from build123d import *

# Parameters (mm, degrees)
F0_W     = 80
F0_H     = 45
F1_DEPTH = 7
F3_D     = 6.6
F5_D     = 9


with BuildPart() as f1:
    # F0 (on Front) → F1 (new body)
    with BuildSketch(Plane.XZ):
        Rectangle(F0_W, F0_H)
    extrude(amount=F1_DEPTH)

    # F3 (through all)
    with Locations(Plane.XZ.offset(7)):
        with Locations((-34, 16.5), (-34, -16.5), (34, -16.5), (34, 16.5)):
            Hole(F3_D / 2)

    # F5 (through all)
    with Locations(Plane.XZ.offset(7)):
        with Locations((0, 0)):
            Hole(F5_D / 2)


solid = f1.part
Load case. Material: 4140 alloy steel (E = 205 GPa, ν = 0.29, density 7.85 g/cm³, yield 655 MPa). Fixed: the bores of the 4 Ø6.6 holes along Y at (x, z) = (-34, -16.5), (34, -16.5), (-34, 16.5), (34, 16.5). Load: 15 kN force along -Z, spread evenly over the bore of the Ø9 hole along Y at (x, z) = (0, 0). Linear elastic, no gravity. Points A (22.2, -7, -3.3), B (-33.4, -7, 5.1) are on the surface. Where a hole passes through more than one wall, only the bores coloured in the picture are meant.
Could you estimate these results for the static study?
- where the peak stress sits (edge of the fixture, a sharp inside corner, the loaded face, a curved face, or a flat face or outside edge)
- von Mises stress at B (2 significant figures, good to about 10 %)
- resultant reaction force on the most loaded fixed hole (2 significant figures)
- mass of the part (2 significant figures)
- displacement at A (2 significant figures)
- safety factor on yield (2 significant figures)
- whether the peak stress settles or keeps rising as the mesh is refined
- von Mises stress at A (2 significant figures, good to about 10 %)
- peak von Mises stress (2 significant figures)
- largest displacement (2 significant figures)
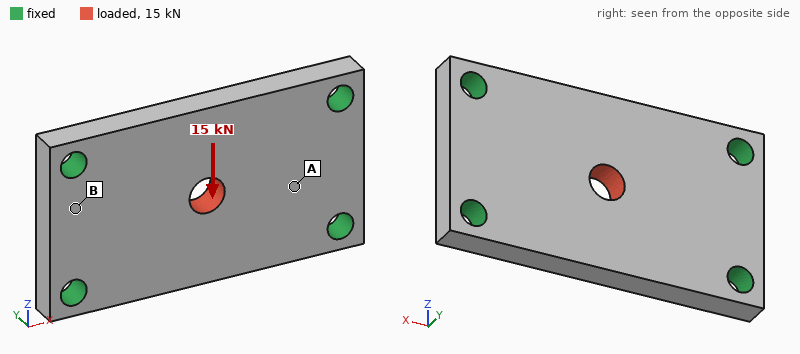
the loaded face
21 MPa
5.1 kN
190 g
4.4 µm
4.9
settles
52 MPa
130 MPa
14 µm
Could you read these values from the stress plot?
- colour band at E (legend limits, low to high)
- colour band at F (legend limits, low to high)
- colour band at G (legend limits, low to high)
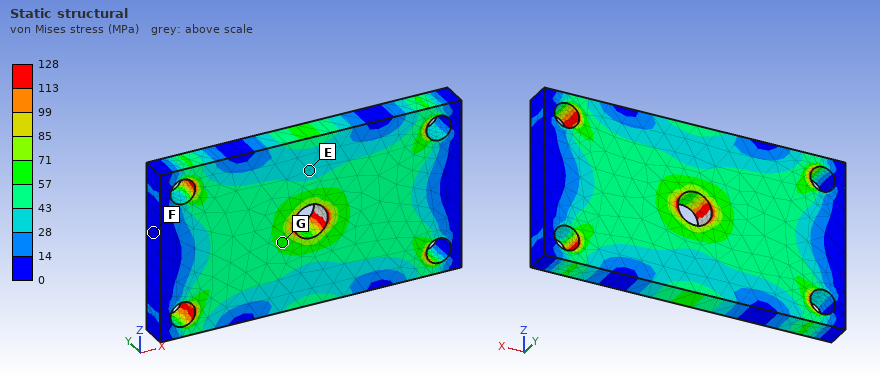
28 to 43 MPa
0 to 14 MPa
57 to 71 MPa
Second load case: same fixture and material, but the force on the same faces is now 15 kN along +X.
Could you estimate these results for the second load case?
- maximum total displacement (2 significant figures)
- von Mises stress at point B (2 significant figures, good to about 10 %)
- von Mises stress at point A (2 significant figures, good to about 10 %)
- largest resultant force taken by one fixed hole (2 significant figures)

6.9 µm
12 MPa
24 MPa
3.9 kN
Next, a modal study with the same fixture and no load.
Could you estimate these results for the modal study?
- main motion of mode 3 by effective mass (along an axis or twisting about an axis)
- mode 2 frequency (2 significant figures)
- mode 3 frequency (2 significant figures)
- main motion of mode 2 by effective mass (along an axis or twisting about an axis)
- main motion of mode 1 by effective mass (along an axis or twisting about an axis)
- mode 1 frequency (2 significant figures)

twisting about Z
11 kHz
19 kHz
twisting about X
along Y
7600 Hz
